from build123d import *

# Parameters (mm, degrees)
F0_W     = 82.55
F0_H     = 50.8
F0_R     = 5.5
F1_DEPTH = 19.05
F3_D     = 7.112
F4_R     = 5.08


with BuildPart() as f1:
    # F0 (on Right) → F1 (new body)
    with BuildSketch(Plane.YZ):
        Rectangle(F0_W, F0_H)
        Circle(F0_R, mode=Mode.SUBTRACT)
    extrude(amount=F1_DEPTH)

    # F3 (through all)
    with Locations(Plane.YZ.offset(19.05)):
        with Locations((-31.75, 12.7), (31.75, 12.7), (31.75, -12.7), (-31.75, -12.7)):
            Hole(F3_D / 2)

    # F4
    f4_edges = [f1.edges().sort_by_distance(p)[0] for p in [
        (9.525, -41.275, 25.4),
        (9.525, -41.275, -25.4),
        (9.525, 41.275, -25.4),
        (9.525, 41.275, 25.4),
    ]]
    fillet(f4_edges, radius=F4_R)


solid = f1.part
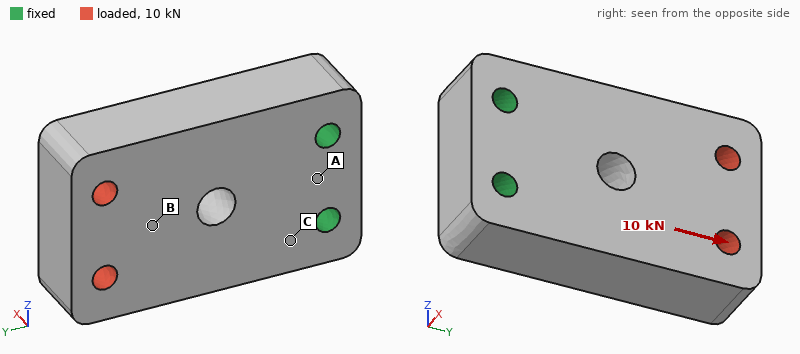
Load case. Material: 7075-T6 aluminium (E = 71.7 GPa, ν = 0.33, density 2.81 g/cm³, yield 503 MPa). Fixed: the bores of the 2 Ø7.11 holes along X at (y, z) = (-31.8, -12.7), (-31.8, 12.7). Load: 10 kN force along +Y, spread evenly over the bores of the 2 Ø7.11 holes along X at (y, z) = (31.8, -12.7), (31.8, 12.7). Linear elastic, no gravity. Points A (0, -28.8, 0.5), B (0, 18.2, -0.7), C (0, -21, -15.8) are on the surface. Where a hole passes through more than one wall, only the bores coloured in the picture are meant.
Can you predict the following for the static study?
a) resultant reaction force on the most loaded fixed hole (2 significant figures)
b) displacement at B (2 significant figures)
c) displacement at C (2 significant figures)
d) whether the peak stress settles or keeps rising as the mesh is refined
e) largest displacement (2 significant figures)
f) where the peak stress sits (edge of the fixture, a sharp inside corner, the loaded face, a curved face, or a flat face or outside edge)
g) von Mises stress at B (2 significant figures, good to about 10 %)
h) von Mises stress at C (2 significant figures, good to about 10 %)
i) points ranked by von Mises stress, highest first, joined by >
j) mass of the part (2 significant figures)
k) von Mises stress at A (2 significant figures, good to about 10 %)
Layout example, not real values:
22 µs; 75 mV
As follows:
5.0 kN; 9.0 µm; 2.1 µm; keeps rising; 13 µm; edge of the fixture; 8.1 MPa; 13 MPa; C > B > A; 210 g; 3.5 MPa
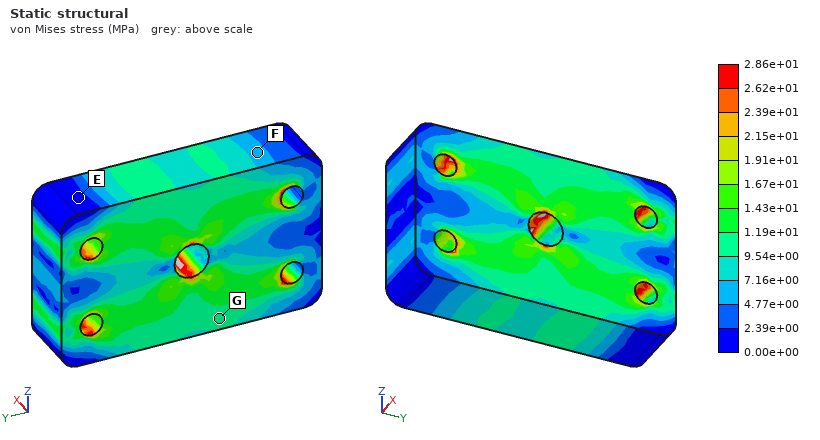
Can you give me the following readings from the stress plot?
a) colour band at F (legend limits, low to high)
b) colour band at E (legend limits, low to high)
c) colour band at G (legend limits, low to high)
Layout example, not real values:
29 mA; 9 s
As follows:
4.77e+00 to 7.16e+00 MPa; 0.00e+00 to 2.39e+00 MPa; 9.54e+00 to 1.19e+01 MPa
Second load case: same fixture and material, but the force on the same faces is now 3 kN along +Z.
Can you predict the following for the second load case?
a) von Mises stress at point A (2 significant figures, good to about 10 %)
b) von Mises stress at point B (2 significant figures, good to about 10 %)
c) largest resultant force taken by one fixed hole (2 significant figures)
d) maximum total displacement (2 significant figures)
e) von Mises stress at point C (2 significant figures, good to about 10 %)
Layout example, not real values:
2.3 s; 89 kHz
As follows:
4.9 MPa; 9.7 MPa; 6.3 kN; 39 µm; 15 MPa
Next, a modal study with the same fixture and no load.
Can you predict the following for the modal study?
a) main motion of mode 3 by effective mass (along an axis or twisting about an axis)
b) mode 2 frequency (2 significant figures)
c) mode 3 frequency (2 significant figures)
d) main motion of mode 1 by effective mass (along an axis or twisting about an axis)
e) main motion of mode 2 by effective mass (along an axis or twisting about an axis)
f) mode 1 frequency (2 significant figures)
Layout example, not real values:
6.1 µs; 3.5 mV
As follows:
twisting about Y; 5400 Hz; 7100 Hz; along X; along Z; 2800 Hz
